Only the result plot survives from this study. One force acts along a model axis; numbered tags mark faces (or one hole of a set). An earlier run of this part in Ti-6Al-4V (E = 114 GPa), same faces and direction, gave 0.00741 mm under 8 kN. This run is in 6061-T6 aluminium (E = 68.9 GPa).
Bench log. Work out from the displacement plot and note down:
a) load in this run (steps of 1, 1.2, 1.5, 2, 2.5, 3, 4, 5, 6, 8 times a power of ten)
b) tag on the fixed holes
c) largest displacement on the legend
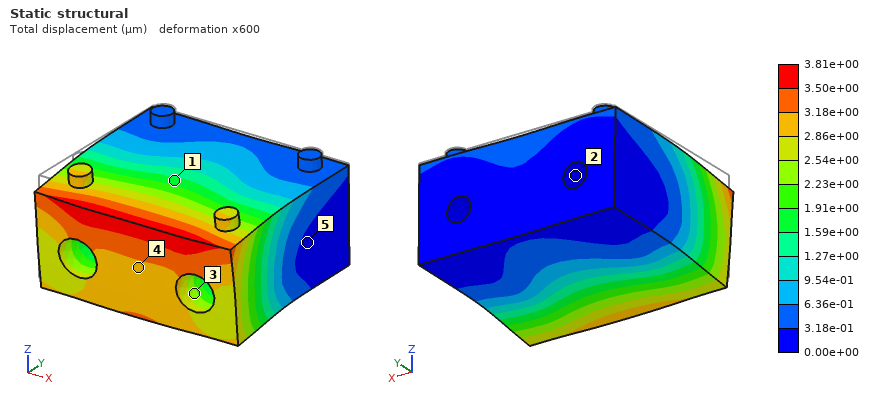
2.5 kN
2
3.81e+00 µm
